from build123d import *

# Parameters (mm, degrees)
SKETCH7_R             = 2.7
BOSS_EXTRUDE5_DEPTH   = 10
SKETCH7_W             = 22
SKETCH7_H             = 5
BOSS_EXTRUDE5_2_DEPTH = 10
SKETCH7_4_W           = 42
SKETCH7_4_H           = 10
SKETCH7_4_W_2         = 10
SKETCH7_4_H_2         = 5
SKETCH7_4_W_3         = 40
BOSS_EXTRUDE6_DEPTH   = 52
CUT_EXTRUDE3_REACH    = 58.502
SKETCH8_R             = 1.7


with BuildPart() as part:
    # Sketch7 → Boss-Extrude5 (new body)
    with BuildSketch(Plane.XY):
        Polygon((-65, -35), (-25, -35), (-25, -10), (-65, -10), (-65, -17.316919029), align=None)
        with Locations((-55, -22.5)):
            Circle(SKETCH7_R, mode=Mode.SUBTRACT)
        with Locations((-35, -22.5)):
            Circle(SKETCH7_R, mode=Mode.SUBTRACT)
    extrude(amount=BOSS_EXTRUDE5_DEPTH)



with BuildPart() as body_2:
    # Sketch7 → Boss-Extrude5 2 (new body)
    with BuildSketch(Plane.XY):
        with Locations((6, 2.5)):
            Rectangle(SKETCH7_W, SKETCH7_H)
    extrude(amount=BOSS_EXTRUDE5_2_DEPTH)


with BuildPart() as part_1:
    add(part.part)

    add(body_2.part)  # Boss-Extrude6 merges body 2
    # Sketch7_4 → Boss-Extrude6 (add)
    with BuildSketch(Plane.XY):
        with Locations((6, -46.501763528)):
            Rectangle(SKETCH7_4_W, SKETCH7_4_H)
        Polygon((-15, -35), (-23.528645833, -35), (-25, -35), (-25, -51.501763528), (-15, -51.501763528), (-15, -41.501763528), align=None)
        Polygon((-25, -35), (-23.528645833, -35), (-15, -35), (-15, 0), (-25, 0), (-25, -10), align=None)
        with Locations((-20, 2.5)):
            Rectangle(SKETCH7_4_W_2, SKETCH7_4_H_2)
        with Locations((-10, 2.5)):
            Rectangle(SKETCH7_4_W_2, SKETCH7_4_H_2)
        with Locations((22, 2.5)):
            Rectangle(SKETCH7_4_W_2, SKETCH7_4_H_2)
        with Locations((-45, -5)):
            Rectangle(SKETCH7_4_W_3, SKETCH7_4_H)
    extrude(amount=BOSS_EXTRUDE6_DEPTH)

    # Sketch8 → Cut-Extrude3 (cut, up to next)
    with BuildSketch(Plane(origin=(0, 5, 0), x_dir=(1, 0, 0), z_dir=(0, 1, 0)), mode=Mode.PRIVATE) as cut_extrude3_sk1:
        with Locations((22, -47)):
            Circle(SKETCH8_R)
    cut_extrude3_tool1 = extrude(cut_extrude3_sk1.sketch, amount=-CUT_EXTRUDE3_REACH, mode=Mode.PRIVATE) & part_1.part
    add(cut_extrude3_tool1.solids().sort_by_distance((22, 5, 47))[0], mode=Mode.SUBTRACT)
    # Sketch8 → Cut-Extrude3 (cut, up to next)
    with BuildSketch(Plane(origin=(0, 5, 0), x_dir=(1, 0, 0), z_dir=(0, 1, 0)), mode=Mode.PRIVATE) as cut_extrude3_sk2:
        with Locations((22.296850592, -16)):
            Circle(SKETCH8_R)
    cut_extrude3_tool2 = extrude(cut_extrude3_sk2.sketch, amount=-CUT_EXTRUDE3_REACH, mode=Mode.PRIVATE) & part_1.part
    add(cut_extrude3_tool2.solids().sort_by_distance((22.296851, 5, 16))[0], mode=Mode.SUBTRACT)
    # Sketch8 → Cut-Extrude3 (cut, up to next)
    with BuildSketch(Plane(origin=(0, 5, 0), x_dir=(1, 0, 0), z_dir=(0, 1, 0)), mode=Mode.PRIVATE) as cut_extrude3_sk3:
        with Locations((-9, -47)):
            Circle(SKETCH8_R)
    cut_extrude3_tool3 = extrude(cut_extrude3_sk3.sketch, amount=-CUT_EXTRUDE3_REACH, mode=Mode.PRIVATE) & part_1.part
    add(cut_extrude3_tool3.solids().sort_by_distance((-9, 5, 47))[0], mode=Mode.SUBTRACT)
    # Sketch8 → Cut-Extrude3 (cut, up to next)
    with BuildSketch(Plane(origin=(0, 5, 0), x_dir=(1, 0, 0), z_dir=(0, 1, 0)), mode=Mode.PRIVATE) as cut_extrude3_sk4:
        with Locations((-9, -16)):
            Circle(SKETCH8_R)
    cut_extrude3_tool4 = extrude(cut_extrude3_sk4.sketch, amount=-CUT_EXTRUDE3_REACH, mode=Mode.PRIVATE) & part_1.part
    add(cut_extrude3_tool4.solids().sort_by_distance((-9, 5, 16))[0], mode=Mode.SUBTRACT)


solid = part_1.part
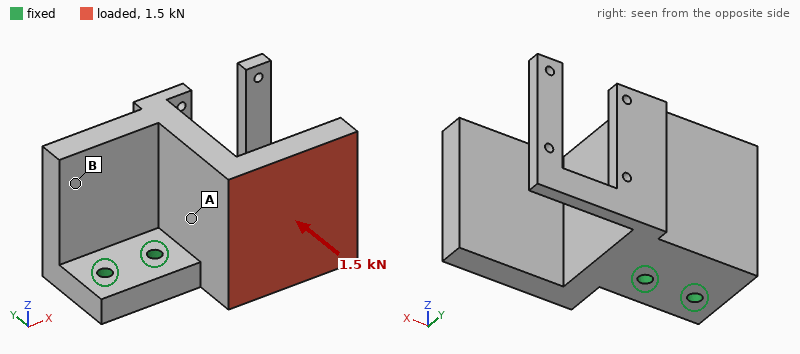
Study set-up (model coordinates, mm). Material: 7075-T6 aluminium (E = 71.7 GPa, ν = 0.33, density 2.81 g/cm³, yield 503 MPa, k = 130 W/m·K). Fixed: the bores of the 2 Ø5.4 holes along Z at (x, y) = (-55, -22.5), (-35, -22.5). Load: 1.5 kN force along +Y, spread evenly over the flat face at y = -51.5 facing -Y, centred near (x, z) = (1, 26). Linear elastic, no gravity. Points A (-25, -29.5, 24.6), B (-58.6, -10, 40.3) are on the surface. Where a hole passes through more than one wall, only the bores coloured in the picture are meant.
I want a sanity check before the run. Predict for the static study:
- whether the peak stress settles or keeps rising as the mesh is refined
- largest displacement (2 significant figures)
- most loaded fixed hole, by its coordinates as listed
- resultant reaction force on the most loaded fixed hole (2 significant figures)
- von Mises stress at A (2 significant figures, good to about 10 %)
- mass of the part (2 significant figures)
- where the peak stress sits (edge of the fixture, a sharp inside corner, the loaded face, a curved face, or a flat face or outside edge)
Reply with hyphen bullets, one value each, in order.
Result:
- keeps rising
- 0.27 mm
- (-35, -22.5)
- 3.5 kN
- 22 MPa
- 250 g
- edge of the fixture
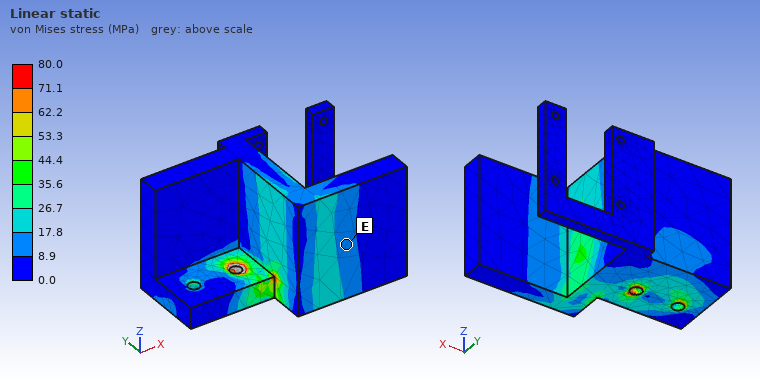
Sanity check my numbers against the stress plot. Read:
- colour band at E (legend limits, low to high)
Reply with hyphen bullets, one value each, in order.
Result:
- 8.9 to 17.8 MPa
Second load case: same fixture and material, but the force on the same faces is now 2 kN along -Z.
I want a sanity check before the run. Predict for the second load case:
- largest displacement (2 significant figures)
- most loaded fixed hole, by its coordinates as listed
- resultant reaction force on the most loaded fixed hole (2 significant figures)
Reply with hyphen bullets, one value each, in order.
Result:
- 0.28 mm
- (-35, -22.5)
- 3.9 kN
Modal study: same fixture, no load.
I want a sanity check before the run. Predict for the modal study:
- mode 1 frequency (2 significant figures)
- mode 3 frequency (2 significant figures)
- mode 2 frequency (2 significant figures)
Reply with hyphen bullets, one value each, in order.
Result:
- 850 Hz
- 1600 Hz
- 1400 Hz
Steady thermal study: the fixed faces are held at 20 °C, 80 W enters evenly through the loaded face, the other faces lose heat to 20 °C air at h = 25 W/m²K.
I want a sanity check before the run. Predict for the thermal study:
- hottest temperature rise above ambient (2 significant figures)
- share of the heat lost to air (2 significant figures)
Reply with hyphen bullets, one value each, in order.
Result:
- 69 K
- 17 %
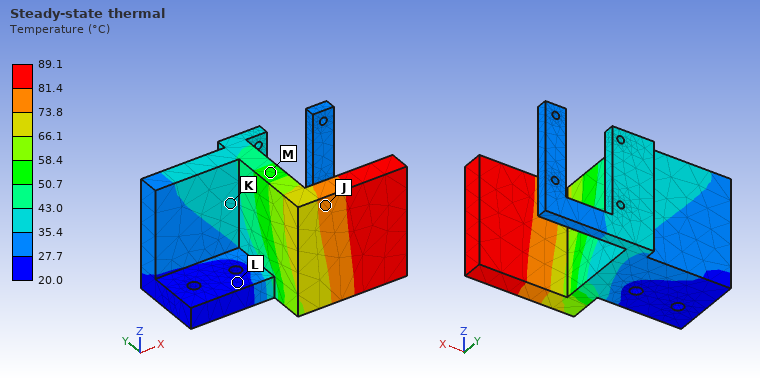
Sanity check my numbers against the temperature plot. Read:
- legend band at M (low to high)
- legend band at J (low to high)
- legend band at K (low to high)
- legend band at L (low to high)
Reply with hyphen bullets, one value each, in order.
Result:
- 50.7 to 58.4 °C
- 73.8 to 81.4 °C
- 35.4 to 43.0 °C
- 20.0 to 27.7 °C
